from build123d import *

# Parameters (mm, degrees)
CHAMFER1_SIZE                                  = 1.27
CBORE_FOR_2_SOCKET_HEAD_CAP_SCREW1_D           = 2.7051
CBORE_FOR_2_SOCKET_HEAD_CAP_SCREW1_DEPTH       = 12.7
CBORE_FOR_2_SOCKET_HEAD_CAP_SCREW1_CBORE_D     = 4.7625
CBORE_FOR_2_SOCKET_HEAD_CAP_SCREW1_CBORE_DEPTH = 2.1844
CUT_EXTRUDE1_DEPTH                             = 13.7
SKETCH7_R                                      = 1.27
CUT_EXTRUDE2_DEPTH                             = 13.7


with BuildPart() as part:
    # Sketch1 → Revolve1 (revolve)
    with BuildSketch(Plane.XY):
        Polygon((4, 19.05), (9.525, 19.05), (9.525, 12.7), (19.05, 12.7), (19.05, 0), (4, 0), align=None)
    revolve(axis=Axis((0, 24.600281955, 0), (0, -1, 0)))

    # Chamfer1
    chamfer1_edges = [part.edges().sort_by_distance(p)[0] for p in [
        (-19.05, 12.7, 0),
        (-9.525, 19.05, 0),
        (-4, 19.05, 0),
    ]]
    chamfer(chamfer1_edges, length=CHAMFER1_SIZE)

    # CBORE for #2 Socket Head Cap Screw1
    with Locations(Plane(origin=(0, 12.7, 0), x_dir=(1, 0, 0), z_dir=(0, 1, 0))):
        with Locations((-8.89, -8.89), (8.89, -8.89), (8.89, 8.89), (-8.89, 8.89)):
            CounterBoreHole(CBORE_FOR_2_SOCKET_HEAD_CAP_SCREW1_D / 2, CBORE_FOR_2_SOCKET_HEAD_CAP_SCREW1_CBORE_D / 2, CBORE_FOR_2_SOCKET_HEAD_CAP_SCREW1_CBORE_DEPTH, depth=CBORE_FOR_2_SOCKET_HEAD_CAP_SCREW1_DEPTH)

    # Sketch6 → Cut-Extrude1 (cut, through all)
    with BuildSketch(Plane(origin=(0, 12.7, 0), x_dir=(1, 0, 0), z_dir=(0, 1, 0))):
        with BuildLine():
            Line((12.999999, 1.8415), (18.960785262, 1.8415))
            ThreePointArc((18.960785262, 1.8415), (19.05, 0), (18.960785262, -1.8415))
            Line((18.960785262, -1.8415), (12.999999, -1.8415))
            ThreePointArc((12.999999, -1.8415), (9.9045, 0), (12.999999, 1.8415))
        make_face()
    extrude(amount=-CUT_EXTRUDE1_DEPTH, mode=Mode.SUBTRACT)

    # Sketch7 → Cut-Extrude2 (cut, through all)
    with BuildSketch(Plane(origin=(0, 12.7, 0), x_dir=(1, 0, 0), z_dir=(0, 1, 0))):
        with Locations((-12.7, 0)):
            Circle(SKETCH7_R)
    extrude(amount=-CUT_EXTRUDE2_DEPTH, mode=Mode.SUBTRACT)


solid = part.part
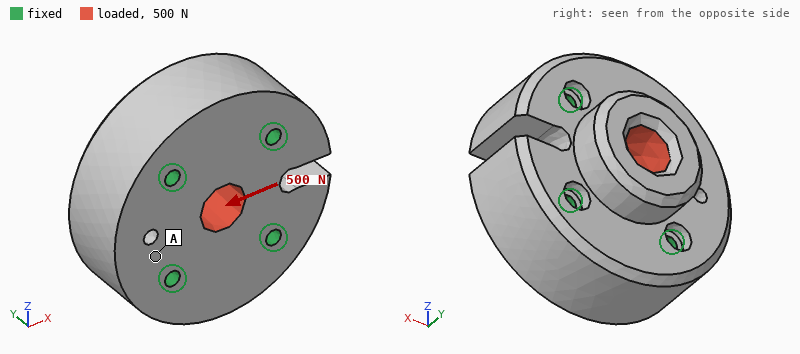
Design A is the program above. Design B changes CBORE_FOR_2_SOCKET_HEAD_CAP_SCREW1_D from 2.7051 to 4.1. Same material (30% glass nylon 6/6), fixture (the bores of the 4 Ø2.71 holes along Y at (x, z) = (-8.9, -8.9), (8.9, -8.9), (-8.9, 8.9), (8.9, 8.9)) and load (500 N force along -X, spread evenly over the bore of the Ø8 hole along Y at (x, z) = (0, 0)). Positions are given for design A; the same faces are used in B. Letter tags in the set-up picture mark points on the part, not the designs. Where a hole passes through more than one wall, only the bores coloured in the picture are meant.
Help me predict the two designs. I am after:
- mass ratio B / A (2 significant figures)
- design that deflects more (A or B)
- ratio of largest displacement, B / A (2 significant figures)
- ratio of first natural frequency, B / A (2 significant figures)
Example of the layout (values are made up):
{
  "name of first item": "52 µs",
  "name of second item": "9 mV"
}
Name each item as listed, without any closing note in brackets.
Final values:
{
  "mass ratio B / A": "0.98",
  "design that deflects more": "A",
  "ratio of largest displacement, B / A": "0.88",
  "ratio of first natural frequency, B / A": "1.2"
}
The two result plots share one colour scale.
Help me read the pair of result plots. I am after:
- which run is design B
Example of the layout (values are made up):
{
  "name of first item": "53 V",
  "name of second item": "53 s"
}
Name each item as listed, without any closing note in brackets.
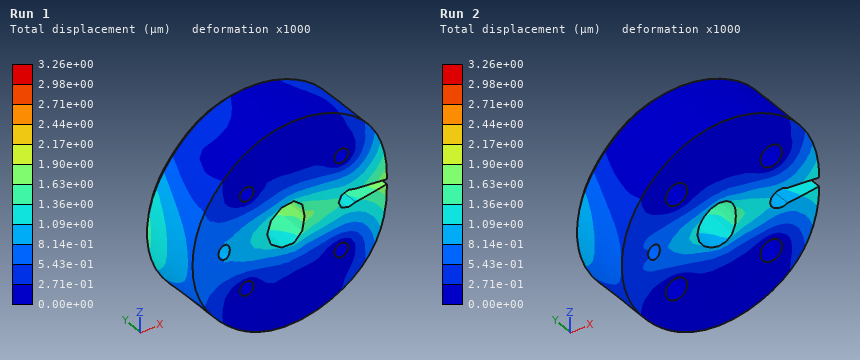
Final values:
{
  "which run is design B": "Run 2"
}
